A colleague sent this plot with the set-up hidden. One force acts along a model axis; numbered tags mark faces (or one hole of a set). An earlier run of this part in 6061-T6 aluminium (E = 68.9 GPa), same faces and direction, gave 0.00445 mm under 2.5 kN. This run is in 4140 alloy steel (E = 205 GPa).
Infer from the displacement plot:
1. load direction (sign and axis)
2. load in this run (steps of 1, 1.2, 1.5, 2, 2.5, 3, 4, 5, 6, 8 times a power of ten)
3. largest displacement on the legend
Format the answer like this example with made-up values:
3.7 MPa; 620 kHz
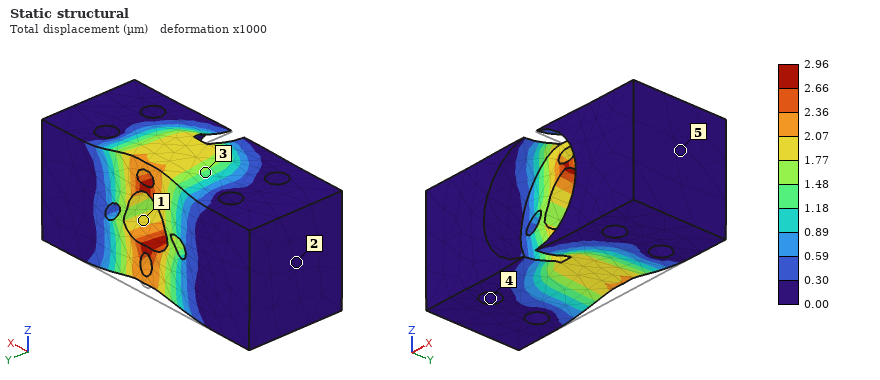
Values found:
+Z; 5 kN; 2.96 µm
